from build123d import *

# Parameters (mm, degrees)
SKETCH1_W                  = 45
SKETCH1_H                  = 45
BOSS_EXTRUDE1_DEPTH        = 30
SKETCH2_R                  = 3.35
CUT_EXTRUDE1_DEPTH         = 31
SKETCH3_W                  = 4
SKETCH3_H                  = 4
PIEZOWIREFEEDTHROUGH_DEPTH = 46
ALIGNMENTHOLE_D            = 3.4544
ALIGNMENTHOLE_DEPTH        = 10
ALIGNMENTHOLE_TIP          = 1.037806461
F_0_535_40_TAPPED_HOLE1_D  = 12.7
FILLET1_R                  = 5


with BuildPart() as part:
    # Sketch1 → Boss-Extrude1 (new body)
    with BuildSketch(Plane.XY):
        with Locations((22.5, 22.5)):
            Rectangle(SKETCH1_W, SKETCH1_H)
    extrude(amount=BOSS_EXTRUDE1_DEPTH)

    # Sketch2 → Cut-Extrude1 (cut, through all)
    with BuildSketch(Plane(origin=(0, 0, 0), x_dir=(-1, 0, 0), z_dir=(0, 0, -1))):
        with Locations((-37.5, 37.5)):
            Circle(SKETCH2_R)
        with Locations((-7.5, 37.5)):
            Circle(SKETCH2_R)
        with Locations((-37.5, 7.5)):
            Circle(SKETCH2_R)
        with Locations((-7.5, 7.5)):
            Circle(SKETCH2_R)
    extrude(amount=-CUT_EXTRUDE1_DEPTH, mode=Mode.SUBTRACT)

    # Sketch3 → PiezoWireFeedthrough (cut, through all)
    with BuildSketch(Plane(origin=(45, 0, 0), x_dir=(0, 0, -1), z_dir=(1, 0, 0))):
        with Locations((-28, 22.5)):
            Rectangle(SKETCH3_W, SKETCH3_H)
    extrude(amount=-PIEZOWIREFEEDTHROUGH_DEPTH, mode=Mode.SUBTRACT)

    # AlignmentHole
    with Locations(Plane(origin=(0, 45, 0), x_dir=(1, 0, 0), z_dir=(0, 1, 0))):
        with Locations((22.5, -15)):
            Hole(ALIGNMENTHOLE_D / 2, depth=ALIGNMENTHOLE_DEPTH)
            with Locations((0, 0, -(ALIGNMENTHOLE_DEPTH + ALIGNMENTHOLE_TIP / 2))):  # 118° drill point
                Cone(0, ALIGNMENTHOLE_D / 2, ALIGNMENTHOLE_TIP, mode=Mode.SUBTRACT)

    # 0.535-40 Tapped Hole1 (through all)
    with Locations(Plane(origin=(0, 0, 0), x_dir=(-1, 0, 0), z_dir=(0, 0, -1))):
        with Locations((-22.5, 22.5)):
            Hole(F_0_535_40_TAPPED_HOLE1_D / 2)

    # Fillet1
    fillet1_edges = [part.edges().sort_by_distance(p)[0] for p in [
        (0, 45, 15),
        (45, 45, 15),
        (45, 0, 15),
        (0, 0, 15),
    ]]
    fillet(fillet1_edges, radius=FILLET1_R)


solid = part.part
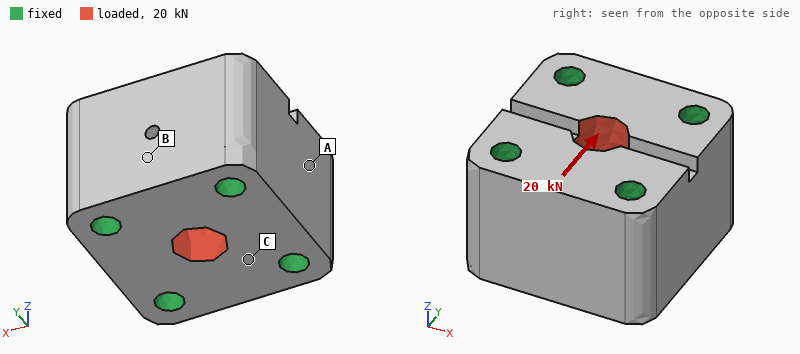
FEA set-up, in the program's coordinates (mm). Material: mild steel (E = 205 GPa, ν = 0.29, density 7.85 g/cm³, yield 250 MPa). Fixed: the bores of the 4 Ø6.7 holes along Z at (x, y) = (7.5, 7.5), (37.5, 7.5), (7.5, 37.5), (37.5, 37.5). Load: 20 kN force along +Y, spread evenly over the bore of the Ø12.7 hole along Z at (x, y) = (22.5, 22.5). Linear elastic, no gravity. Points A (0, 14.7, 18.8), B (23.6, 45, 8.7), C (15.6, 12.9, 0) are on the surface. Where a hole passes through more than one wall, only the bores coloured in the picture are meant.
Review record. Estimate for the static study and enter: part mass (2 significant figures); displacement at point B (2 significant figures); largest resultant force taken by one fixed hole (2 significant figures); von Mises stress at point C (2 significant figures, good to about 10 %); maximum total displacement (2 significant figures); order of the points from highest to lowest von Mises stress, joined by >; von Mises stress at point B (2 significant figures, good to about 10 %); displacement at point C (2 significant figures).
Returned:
400 g
0.86 µm
5.4 kN
16 MPa
1.6 µm
C > B > A
11 MPa
0.80 µm
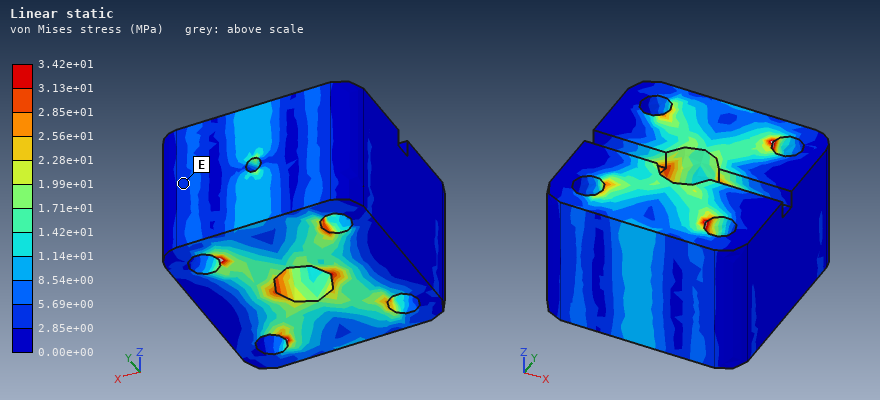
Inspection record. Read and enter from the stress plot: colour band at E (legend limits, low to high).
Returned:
2.85e+00 to 5.69e+00 MPa
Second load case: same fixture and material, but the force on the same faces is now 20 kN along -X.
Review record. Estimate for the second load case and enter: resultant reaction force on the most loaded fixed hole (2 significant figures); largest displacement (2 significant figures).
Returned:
5.5 kN
1.6 µm
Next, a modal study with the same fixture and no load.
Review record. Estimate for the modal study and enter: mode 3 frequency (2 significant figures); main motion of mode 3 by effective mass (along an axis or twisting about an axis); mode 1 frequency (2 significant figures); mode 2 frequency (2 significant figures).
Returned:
54 kHz
along Y
48 kHz
48 kHz
